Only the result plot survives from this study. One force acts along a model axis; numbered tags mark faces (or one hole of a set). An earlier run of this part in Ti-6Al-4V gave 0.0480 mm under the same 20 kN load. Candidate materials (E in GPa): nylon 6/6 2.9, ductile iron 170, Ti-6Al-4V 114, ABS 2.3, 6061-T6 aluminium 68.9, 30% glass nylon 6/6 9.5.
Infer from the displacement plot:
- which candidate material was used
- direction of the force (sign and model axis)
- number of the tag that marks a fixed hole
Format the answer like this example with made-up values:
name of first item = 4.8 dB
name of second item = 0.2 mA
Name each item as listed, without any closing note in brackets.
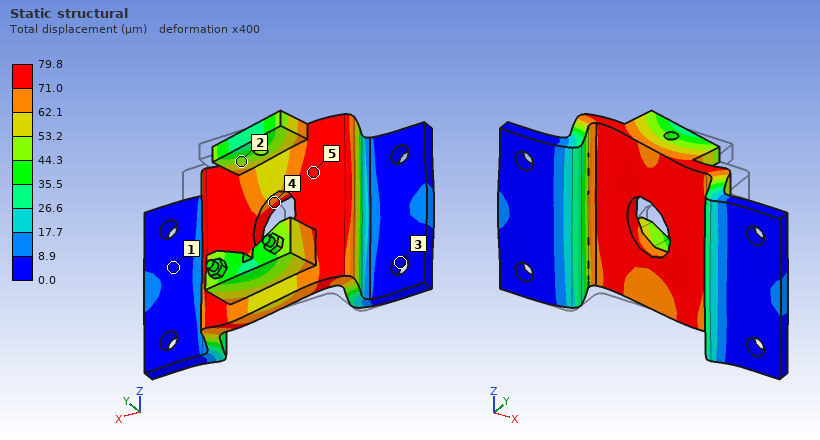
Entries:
which candidate material was used = 6061-T6 aluminium
direction of the force = -X
number of the tag that marks a fixed hole = 3
